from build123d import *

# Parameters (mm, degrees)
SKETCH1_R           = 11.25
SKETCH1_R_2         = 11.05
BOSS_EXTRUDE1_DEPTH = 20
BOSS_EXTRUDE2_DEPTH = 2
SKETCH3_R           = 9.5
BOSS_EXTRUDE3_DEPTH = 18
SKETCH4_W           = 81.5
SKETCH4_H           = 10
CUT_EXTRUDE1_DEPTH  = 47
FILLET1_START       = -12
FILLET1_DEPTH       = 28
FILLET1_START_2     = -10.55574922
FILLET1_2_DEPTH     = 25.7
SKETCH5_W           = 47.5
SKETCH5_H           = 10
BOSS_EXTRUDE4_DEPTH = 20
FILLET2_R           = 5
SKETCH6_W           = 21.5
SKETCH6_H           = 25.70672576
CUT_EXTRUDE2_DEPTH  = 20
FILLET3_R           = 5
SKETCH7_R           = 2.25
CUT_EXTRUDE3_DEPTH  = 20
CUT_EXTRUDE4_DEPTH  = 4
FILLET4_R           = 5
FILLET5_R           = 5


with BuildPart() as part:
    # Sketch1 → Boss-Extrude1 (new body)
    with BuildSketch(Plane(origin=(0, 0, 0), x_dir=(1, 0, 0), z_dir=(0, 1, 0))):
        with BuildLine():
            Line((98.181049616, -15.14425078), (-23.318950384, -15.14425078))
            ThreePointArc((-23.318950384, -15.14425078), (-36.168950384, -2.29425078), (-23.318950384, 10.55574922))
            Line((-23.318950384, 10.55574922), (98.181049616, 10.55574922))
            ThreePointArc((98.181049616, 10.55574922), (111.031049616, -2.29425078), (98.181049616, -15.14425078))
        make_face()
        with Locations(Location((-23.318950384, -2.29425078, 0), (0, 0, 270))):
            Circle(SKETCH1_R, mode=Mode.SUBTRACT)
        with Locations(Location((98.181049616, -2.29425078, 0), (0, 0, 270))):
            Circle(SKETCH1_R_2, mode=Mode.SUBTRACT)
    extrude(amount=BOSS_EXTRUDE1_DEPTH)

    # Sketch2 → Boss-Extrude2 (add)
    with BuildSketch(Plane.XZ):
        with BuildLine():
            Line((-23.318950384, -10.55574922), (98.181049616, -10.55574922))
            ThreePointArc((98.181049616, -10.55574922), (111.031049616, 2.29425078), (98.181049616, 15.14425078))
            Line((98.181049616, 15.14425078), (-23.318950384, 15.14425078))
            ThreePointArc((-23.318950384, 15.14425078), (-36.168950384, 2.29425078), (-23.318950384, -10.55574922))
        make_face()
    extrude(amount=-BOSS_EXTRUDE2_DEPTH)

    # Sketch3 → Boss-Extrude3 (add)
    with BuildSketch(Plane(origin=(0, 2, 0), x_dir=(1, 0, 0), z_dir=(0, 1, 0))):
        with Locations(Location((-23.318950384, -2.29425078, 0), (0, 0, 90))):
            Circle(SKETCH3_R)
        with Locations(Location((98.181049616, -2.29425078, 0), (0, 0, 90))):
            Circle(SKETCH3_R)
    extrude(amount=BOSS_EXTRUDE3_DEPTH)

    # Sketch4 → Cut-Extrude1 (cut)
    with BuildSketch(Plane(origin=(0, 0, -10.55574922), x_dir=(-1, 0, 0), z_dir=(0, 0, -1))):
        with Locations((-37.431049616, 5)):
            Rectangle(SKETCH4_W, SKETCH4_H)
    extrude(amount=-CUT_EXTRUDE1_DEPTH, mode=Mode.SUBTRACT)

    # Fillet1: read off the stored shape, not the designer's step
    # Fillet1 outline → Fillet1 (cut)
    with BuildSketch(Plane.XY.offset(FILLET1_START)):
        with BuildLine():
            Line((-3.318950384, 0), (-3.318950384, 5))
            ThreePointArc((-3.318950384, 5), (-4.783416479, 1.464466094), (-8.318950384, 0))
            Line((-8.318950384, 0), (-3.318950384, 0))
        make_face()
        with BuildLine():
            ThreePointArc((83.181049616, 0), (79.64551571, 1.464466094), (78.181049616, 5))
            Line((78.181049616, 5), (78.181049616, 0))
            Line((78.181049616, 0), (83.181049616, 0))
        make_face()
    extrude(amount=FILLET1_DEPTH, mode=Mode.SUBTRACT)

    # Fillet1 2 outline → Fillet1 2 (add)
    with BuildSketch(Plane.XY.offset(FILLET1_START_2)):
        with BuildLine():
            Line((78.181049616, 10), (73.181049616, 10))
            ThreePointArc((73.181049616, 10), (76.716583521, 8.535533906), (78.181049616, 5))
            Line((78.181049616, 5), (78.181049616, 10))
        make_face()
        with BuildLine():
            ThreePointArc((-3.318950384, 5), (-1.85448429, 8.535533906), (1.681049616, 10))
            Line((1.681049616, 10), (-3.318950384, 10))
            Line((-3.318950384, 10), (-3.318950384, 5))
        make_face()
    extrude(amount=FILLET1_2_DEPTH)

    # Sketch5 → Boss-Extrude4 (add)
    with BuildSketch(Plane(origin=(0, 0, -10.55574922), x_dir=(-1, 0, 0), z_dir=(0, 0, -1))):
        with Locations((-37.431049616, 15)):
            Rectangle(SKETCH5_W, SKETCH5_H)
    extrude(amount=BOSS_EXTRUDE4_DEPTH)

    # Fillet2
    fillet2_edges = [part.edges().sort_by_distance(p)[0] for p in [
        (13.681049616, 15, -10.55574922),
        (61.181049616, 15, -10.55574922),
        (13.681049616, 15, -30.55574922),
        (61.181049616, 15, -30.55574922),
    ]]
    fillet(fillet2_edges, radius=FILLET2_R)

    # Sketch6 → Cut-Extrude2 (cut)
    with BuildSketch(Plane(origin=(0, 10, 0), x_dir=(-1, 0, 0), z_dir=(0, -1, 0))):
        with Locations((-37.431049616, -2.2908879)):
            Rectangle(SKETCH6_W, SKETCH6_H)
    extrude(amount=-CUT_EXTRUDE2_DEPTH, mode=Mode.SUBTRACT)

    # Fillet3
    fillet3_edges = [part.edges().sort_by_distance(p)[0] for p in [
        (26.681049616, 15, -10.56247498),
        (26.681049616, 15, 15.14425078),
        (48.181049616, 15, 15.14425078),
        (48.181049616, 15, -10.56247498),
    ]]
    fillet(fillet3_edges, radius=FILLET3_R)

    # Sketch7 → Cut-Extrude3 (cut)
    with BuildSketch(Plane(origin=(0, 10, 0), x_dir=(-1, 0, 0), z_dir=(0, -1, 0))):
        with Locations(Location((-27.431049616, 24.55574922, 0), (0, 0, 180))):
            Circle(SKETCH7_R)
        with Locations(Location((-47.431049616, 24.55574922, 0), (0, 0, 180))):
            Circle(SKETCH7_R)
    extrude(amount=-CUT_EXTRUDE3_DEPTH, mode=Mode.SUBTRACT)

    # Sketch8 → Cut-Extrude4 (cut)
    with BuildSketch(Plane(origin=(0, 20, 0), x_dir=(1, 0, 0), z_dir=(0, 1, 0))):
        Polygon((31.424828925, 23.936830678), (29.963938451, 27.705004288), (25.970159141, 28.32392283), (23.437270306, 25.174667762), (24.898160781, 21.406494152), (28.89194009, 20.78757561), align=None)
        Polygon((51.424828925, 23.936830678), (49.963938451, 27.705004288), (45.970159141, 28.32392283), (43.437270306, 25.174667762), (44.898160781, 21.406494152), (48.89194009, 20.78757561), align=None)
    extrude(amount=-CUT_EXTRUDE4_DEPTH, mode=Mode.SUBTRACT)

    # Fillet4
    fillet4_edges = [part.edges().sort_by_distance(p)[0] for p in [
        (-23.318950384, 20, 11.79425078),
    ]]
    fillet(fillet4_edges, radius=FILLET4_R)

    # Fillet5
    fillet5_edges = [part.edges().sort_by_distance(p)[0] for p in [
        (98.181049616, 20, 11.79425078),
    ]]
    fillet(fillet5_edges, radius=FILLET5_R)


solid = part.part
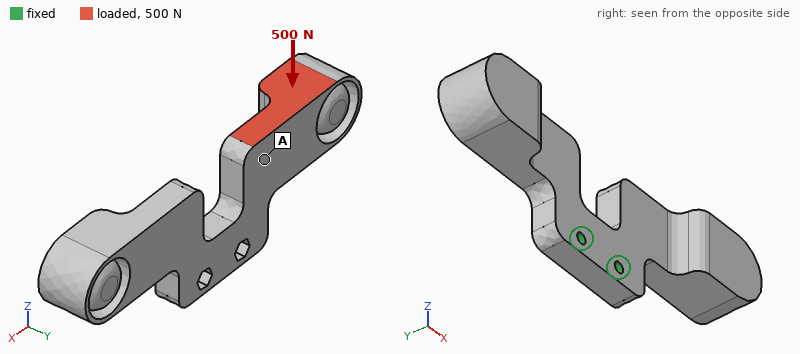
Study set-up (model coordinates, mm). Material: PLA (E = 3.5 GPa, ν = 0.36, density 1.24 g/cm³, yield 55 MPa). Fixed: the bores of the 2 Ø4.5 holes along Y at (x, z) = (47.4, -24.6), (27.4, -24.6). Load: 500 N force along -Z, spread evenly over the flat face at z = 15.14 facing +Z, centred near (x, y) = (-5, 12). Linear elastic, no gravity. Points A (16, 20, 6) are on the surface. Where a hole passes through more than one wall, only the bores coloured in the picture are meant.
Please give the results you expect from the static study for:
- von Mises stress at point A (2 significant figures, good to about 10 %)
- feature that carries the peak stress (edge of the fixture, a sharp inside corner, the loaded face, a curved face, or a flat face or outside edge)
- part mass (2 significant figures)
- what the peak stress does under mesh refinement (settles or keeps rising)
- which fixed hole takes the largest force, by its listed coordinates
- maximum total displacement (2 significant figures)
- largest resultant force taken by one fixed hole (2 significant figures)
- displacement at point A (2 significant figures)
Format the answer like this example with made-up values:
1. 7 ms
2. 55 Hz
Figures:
1. 6.5 MPa
2. edge of the fixture
3. 63 g
4. keeps rising
5. (27.4, -24.6)
6. 1.9 mm
7. 1.2 kN
8. 0.56 mm
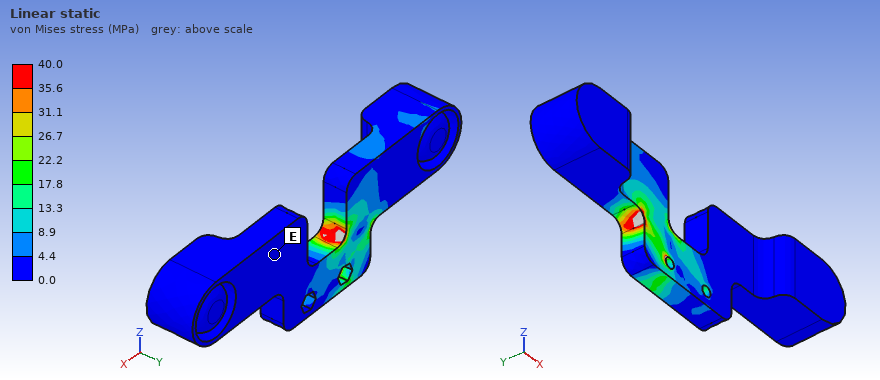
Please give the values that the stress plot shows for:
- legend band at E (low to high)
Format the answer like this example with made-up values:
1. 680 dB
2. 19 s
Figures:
1. 0.0 to 4.4 MPa
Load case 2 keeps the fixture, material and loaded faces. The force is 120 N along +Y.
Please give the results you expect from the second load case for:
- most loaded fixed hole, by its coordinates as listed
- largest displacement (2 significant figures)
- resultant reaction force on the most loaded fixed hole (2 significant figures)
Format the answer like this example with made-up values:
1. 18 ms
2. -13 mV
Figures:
1. (27.4, -24.6)
2. 1.8 mm
3. 250 N
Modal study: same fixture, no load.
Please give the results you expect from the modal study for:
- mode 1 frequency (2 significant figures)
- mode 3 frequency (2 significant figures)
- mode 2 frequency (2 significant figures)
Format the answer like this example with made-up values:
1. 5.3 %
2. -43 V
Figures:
1. 320 Hz
2. 540 Hz
3. 330 Hz
